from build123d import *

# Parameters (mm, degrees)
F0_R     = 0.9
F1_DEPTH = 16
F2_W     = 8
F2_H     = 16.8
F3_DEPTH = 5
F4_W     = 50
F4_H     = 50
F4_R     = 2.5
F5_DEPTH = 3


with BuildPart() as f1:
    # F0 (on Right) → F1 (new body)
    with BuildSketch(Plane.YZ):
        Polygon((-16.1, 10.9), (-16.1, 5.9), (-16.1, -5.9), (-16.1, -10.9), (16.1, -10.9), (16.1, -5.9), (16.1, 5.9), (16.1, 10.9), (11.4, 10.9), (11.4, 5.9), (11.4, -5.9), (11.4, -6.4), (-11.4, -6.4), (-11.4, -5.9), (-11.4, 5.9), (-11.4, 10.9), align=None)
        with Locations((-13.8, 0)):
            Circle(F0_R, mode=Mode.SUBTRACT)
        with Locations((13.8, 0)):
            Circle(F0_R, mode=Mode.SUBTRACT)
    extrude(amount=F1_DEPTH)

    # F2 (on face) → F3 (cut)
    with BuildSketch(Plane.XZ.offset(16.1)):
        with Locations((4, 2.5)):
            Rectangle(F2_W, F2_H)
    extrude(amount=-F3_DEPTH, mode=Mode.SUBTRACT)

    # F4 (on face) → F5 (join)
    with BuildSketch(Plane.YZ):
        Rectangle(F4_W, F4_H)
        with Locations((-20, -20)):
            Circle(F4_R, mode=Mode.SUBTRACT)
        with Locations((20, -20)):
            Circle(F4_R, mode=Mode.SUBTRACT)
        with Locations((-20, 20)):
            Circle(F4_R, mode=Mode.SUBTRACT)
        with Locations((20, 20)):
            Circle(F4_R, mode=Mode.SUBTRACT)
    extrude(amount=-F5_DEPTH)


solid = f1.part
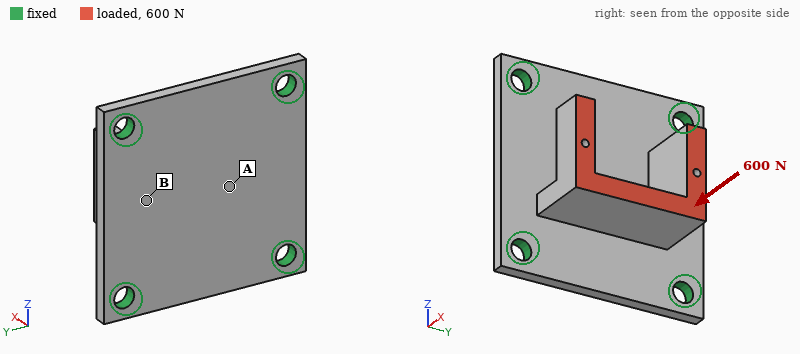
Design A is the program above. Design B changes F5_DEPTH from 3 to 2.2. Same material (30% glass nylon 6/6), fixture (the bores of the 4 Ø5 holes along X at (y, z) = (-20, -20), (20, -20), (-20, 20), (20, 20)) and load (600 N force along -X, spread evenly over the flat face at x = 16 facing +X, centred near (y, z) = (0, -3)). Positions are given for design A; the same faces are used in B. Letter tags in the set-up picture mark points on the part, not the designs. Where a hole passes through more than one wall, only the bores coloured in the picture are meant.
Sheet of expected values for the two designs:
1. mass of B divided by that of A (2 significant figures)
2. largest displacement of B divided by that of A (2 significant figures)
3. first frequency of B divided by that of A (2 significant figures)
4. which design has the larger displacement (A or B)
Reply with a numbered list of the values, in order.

1. 0.83
2. 1.4
3. 0.82
4. B
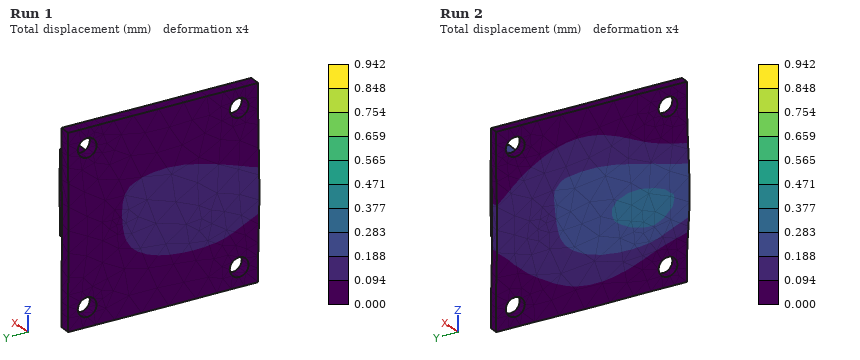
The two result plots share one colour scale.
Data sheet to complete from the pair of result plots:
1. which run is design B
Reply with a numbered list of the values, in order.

1. Run 2
